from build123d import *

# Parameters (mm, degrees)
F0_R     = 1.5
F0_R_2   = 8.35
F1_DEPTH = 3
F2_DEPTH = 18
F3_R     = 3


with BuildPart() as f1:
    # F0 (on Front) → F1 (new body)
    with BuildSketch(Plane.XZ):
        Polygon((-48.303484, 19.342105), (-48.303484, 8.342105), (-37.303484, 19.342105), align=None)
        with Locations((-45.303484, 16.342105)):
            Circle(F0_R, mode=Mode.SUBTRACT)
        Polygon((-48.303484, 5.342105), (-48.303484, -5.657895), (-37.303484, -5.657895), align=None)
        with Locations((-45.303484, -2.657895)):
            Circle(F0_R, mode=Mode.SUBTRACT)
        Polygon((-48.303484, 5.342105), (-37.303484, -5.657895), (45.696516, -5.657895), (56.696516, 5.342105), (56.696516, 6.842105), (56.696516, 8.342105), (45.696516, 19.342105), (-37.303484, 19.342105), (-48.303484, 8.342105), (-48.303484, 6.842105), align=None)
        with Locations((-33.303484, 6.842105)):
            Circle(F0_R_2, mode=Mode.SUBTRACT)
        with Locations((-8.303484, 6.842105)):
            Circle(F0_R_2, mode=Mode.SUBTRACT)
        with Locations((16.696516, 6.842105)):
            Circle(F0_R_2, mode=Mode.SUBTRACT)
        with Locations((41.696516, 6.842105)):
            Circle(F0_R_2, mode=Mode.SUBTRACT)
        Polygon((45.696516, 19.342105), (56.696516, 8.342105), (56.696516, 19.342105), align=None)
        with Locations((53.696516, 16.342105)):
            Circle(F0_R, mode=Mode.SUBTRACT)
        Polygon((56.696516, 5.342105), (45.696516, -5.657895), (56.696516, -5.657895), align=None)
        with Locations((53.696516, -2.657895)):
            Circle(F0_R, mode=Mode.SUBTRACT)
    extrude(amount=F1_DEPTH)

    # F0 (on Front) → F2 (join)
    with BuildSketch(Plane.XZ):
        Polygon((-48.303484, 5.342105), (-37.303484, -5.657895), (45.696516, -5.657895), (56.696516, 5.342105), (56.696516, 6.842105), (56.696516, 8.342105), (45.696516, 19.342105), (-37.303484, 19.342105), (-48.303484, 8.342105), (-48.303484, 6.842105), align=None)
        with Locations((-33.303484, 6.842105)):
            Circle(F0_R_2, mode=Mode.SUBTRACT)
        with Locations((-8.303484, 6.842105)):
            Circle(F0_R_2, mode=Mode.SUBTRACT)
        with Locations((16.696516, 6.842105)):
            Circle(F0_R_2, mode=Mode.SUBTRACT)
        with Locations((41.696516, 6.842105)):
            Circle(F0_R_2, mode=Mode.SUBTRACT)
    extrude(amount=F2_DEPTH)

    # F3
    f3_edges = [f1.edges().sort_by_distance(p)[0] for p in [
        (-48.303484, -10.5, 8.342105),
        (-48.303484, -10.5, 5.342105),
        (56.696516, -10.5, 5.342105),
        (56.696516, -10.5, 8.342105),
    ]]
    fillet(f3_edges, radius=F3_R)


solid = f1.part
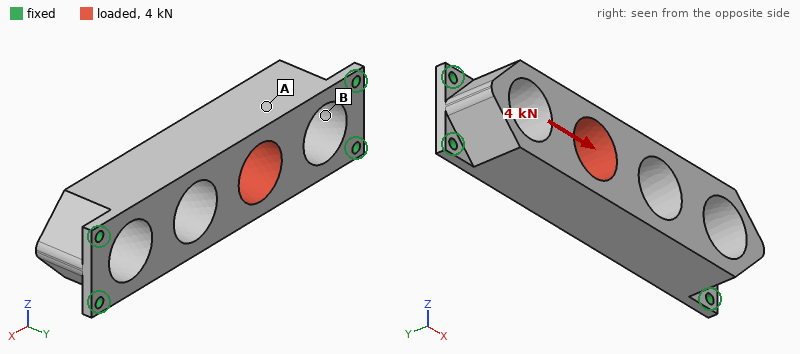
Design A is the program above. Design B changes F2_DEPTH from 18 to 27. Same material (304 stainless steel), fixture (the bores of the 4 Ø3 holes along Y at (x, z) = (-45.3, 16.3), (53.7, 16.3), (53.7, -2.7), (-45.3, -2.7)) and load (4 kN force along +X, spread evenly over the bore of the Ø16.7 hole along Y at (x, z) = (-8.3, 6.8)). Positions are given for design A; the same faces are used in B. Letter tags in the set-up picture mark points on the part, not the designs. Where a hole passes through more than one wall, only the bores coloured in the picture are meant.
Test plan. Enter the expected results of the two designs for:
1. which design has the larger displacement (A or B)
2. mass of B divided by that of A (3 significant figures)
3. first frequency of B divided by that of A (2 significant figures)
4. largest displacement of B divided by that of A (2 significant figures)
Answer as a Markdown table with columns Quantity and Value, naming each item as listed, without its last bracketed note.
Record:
| Quantity | Value |
|---|---|
| which design has the larger displacement | A |
| mass of B divided by that of A | 1.49 |
| first frequency of B divided by that of A | 0.75 |
| largest displacement of B divided by that of A | 0.82 |
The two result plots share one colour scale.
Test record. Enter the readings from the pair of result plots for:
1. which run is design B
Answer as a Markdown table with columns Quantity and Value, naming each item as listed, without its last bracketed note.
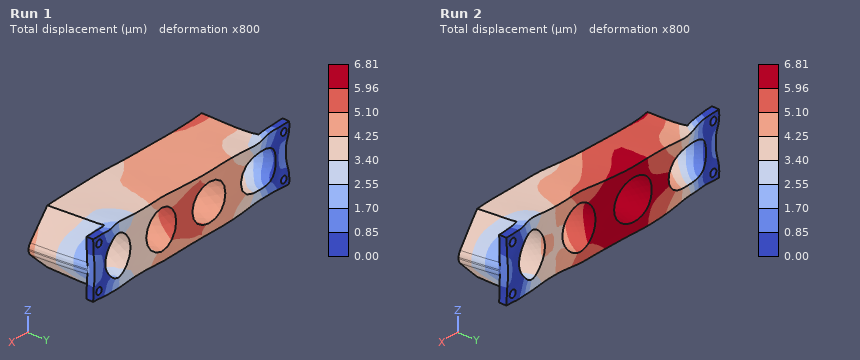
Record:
| Quantity | Value |
|---|---|
| which run is design B | Run 1 |
